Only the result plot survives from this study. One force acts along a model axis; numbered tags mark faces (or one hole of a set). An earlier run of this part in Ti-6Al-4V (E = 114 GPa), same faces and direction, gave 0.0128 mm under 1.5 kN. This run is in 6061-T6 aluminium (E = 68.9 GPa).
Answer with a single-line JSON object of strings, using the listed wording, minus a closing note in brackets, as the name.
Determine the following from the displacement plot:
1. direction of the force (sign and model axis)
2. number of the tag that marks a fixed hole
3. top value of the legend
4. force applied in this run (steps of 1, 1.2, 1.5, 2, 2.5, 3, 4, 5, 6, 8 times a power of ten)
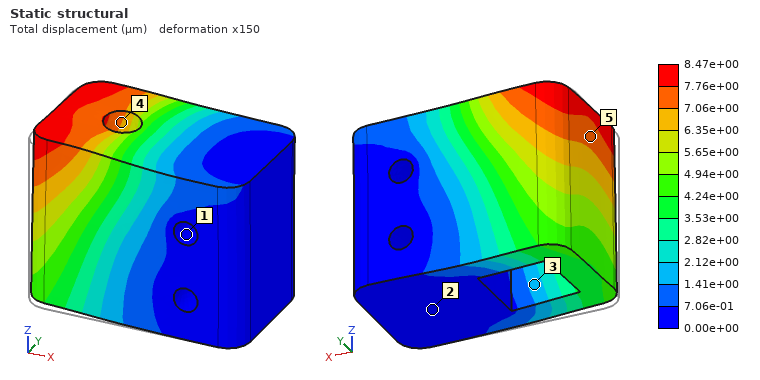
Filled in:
{"direction of the force": "+Y", "number of the tag that marks a fixed hole": "1", "top value of the legend": "8.47e+00 µm", "force applied in this run": "600 N"}
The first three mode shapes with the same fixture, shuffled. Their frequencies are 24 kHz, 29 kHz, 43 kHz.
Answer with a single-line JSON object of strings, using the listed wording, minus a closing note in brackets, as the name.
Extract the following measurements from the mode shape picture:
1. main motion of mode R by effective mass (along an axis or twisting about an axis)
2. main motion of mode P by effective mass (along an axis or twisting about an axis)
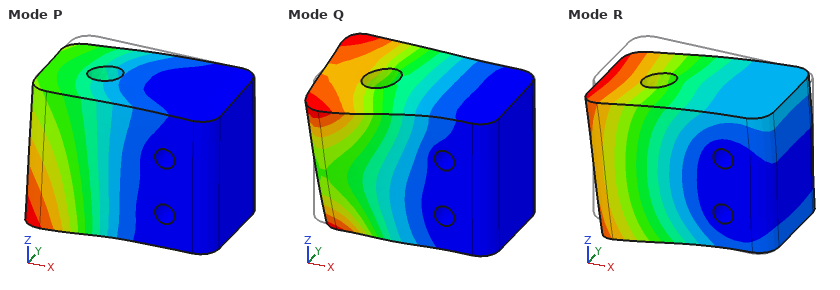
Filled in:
{"main motion of mode R by effective mass": "along Z", "main motion of mode P by effective mass": "along Y"}
